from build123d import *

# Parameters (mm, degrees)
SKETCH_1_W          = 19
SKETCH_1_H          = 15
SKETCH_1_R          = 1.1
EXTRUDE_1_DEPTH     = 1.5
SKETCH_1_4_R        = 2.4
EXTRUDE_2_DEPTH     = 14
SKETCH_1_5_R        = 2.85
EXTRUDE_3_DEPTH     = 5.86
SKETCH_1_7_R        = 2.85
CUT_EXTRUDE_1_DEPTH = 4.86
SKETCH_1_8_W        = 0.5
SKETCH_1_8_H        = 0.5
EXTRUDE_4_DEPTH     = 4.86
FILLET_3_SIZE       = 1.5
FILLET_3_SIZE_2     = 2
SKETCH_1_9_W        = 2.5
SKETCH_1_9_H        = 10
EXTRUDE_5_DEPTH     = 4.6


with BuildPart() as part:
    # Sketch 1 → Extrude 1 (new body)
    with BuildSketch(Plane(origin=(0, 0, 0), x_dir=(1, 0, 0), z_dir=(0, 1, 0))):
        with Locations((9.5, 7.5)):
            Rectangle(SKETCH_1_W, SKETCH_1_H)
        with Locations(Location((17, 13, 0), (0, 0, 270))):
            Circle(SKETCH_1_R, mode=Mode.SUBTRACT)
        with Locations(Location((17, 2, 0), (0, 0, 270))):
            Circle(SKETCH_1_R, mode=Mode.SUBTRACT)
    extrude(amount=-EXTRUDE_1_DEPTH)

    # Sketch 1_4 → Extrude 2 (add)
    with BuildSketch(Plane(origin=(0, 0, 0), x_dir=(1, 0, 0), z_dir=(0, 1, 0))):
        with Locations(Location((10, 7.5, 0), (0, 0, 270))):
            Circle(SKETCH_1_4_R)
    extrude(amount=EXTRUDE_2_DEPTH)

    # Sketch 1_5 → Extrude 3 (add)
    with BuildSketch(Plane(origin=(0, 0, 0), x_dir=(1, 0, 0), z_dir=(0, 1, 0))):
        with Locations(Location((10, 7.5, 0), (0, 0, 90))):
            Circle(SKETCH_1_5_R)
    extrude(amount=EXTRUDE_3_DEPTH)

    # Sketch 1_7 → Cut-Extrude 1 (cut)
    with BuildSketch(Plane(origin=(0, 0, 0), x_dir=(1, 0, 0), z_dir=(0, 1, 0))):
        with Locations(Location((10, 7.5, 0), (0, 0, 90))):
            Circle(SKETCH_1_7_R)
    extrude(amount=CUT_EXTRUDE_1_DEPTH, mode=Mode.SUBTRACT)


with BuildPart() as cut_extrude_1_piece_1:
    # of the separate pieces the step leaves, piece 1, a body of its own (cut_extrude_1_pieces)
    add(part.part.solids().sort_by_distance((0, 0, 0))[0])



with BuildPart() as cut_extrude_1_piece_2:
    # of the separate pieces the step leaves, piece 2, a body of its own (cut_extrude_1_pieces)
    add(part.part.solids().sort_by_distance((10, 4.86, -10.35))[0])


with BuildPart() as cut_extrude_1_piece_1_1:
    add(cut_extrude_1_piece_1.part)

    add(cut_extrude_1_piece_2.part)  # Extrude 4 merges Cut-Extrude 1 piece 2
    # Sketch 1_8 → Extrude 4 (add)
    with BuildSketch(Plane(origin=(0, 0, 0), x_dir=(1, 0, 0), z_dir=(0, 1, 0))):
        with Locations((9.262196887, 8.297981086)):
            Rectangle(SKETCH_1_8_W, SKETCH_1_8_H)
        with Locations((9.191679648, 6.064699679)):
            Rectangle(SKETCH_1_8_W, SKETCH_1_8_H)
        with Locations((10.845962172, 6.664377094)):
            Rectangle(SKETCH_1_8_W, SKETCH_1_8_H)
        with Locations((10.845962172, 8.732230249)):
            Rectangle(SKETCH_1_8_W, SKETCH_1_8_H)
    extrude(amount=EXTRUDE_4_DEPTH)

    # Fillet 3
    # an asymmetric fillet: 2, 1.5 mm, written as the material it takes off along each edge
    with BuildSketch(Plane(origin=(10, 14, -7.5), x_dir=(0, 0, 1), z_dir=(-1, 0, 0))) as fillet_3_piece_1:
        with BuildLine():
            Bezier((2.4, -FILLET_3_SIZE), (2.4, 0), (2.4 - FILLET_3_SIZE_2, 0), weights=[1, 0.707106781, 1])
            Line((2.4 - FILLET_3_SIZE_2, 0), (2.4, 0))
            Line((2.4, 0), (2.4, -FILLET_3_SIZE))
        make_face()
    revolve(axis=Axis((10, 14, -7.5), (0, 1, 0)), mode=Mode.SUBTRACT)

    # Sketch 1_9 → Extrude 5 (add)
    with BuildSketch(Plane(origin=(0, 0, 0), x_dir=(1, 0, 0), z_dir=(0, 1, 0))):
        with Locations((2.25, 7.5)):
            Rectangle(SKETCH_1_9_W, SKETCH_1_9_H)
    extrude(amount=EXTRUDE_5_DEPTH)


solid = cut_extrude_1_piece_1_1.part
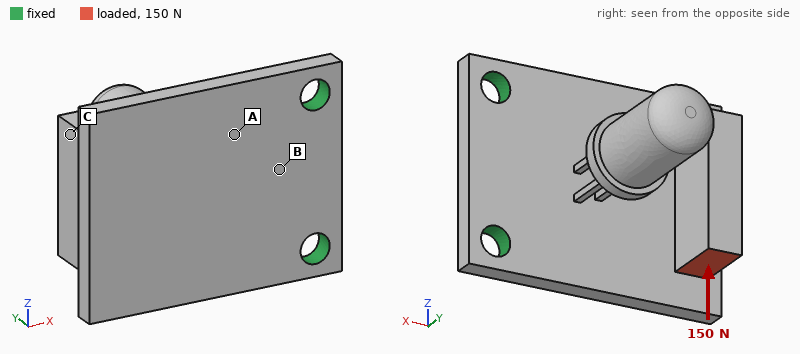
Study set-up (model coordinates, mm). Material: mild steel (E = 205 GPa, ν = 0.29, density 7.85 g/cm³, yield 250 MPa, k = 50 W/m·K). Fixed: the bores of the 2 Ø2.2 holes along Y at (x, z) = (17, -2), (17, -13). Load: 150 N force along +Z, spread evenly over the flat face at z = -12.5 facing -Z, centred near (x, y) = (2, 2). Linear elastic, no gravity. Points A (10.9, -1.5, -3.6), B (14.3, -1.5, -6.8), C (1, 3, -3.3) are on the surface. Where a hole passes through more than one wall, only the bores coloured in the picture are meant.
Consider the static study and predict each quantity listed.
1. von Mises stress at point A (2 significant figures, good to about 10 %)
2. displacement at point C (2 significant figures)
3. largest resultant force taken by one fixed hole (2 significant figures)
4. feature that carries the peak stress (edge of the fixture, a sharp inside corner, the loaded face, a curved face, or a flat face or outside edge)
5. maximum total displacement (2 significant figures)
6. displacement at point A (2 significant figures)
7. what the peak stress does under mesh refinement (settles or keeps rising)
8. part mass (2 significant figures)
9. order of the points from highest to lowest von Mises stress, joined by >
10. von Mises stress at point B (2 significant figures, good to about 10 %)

44 MPa
19 µm
200 N
edge of the fixture
24 µm
3.8 µm
keeps rising
5.5 g
A > B > C
19 MPa
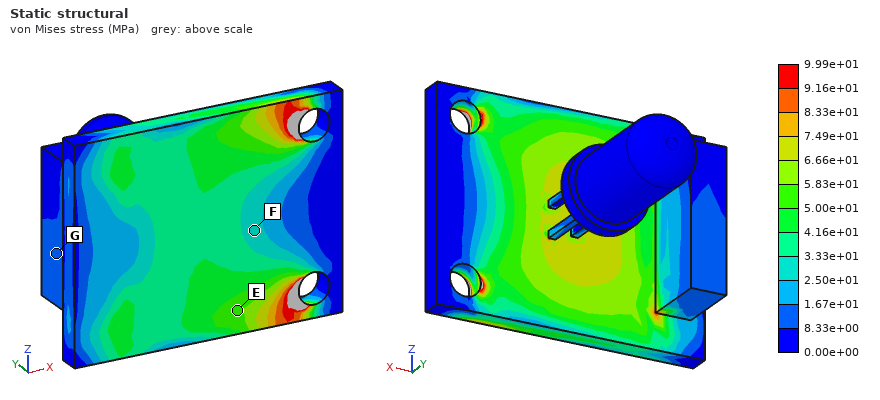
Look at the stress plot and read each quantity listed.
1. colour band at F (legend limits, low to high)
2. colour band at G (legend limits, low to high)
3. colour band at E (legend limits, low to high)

2.50e+01 to 3.33e+01 MPa
8.33e+00 to 1.67e+01 MPa
5.00e+01 to 5.83e+01 MPa
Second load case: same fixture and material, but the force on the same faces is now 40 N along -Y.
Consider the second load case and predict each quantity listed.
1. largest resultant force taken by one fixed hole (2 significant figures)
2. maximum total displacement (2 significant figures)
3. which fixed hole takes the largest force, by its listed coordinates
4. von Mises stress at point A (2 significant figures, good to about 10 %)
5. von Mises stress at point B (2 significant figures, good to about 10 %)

37 N
68 µm
(17, -13)
57 MPa
62 MPa
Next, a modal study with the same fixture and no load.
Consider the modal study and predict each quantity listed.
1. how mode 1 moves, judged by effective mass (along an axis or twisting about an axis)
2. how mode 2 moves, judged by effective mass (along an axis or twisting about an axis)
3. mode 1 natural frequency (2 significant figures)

along X
along Z
1800 Hz
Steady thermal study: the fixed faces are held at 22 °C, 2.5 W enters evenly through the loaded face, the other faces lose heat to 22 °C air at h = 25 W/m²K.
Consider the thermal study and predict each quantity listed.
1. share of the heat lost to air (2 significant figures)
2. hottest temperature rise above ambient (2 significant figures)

15 %
46 K
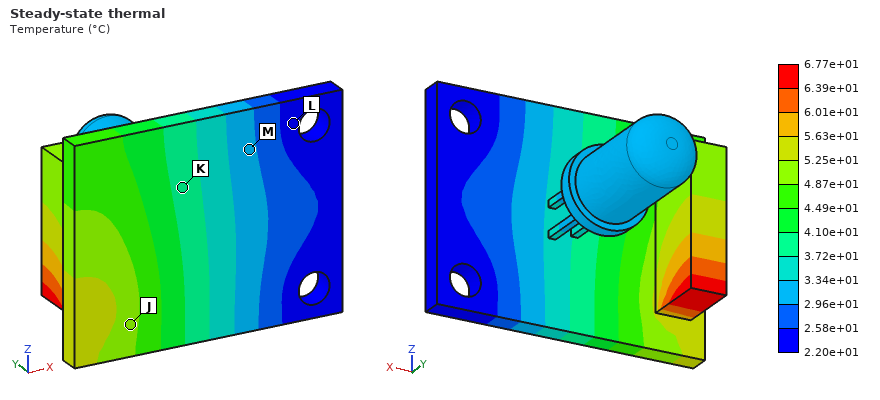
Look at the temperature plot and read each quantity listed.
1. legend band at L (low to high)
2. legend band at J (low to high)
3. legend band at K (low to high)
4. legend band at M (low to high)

2.20e+01 to 2.58e+01 °C
4.87e+01 to 5.25e+01 °C
3.72e+01 to 4.10e+01 °C
2.96e+01 to 3.34e+01 °C
